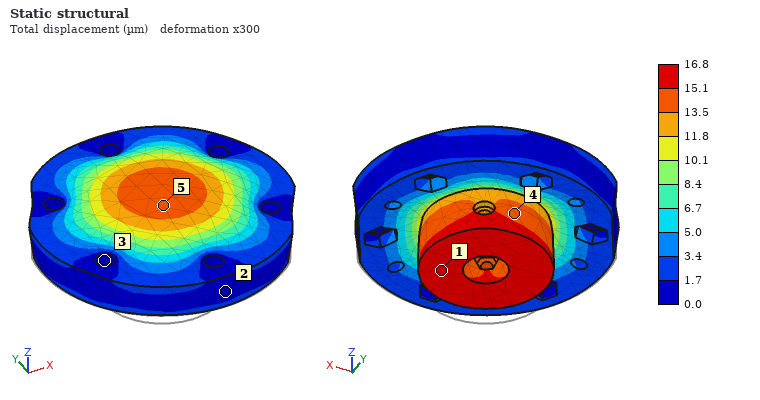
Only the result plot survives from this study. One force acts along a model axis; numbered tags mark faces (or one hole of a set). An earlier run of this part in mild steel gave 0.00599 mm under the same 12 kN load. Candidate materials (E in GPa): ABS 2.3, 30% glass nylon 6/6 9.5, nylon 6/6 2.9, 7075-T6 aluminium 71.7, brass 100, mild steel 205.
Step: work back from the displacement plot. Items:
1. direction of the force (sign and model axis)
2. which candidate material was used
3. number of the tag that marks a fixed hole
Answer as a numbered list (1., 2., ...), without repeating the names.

1. +Z
2. 7075-T6 aluminium
3. 3
